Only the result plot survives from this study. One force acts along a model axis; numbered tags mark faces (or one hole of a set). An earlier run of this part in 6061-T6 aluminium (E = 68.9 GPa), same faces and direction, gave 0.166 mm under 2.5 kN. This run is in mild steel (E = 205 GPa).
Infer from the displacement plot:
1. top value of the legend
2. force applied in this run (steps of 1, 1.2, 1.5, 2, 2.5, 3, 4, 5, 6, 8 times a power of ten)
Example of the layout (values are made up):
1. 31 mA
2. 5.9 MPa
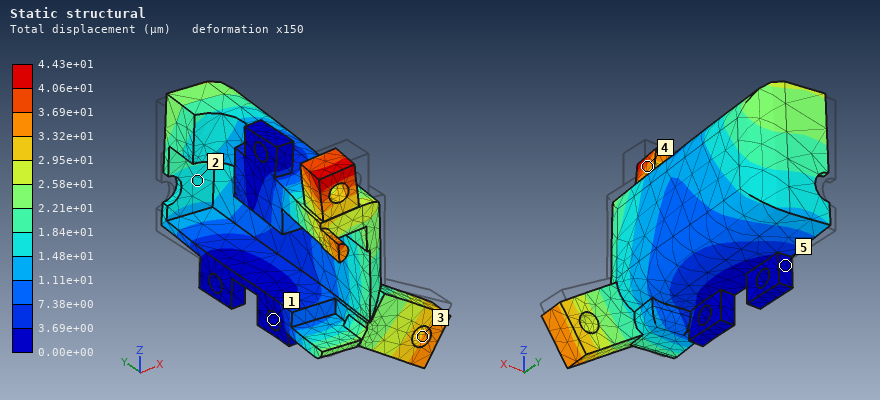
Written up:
1. 4.43e+01 µm
2. 2 kN
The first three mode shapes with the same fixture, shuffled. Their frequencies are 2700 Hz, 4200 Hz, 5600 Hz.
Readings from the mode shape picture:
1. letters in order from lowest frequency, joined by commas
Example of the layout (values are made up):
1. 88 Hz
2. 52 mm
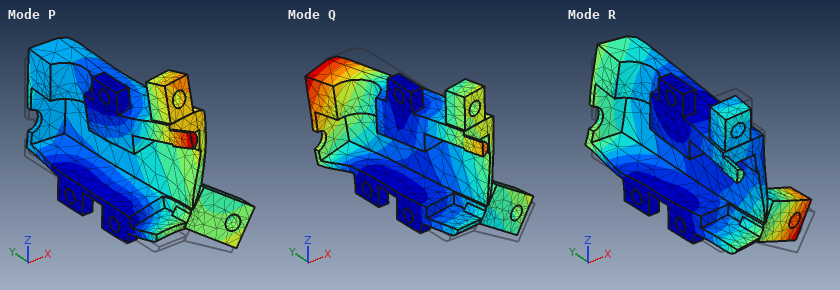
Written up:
1. Q, R, P
